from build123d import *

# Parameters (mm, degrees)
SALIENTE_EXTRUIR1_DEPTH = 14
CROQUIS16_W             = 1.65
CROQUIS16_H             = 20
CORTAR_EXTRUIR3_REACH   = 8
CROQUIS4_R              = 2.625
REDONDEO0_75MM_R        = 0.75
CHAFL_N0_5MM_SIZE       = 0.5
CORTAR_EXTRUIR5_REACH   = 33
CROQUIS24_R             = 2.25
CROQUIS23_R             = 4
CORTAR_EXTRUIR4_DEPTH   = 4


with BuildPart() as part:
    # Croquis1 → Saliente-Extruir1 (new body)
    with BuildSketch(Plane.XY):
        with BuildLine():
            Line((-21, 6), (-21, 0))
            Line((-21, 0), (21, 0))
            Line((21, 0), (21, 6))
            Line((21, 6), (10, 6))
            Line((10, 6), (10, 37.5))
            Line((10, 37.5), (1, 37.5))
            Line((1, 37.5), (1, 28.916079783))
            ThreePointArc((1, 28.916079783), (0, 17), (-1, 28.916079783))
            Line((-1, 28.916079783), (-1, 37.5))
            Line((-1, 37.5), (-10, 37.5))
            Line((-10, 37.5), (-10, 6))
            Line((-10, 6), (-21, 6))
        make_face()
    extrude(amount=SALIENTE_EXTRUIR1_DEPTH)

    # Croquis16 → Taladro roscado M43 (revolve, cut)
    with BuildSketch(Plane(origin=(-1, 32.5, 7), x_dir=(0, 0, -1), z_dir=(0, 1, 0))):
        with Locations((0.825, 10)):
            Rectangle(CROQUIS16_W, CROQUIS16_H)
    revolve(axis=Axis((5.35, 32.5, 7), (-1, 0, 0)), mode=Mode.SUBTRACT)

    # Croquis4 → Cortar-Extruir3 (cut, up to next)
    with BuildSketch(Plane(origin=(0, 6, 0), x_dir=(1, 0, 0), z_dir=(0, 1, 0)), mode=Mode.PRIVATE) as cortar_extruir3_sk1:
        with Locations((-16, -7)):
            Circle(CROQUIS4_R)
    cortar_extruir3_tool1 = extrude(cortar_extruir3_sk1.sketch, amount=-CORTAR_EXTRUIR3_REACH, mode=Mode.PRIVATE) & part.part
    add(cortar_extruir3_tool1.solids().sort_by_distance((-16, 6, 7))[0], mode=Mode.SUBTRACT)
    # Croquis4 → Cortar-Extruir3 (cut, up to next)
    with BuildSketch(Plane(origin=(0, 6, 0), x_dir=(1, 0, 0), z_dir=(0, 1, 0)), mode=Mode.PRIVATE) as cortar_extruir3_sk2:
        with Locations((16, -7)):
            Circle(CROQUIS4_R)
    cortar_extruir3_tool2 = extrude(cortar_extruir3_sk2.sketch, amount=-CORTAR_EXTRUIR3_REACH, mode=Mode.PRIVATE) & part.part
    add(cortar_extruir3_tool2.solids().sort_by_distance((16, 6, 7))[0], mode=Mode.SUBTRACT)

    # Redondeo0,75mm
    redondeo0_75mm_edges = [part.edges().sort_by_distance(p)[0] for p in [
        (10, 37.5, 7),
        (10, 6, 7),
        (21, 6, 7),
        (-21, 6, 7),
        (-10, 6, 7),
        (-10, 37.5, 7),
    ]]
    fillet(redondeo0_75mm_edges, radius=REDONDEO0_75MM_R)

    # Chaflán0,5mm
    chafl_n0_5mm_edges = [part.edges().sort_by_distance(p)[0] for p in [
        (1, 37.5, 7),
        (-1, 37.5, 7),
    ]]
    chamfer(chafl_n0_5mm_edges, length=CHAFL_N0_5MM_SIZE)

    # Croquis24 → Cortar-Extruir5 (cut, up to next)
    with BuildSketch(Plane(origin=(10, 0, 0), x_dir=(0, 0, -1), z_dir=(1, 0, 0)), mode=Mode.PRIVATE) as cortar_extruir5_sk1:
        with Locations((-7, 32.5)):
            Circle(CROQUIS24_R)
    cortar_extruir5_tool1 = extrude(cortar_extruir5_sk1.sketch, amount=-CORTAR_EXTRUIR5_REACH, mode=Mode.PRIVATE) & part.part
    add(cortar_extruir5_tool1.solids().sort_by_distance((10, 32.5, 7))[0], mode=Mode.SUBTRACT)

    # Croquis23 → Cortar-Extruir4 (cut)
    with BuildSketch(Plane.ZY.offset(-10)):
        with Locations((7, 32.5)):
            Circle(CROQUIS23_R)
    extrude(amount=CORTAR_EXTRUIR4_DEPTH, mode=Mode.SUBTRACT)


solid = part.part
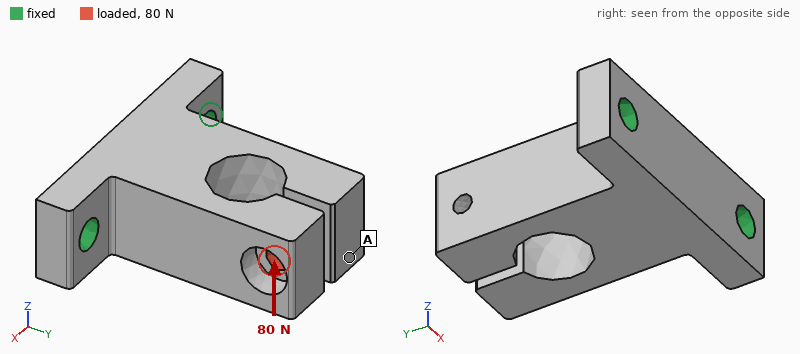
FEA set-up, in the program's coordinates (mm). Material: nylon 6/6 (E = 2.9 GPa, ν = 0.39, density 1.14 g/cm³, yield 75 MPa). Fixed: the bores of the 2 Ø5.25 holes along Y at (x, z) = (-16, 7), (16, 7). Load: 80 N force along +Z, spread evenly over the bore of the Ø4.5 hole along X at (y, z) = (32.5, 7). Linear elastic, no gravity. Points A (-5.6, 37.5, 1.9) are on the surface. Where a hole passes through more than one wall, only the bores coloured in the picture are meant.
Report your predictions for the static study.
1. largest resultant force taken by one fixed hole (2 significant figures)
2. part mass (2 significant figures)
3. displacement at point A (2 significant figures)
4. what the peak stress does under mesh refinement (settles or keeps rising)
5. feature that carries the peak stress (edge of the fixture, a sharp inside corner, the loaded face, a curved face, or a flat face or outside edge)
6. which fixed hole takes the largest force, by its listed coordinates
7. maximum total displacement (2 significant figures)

48 N
11 g
0.29 mm
keeps rising
edge of the fixture
(16, 7)
0.51 mm
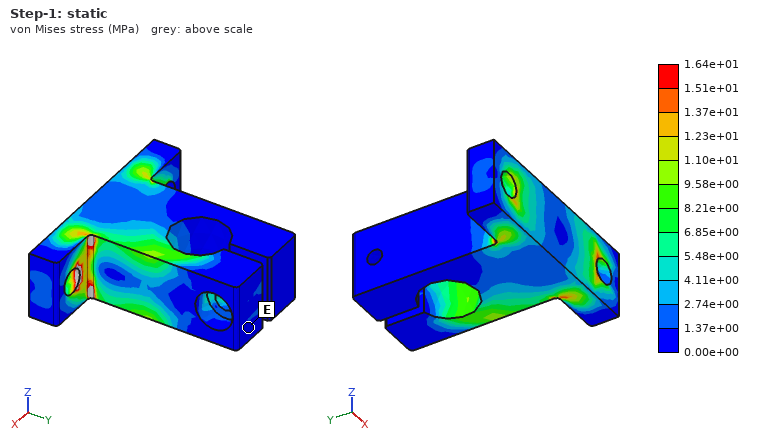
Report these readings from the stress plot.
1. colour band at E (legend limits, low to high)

0.00e+00 to 1.37e+00 MPa
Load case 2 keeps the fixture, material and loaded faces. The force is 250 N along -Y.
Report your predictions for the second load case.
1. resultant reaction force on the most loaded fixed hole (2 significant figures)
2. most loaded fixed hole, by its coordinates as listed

170 N
(16, 7)
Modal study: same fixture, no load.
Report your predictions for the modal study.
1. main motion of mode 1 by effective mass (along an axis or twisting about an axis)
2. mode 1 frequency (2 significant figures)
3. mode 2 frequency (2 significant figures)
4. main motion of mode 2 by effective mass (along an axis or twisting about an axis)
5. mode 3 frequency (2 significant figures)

along Z
1400 Hz
1800 Hz
along X
2000 Hz
